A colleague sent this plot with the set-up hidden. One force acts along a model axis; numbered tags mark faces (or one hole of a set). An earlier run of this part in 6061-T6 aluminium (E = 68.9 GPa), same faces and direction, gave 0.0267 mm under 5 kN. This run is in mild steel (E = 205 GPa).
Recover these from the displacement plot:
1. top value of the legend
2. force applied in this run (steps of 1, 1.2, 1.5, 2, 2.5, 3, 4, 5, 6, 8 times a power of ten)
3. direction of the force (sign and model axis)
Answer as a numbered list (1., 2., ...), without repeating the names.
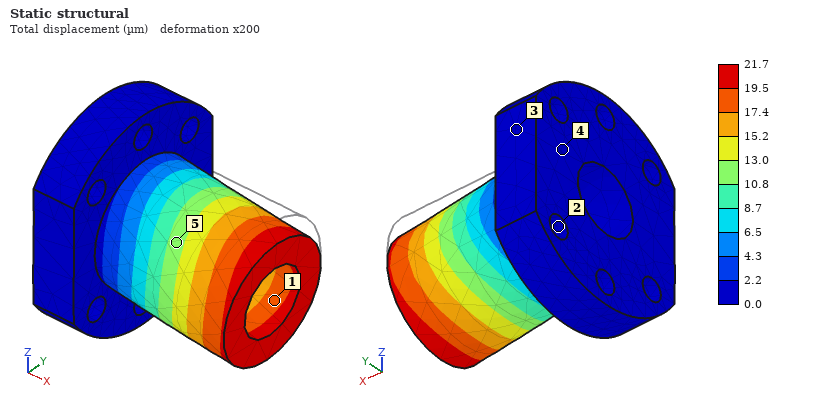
1. 21.7 µm
2. 12 kN
3. -Z
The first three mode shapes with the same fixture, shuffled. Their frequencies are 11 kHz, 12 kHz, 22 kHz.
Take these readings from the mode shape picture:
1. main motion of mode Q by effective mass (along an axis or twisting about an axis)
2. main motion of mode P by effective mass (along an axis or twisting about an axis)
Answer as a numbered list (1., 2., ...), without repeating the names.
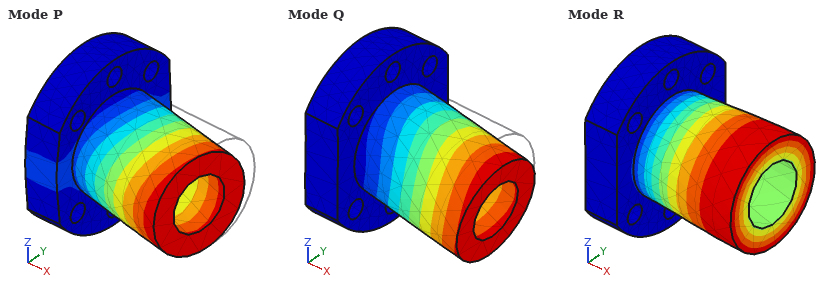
1. along Z
2. along Y
